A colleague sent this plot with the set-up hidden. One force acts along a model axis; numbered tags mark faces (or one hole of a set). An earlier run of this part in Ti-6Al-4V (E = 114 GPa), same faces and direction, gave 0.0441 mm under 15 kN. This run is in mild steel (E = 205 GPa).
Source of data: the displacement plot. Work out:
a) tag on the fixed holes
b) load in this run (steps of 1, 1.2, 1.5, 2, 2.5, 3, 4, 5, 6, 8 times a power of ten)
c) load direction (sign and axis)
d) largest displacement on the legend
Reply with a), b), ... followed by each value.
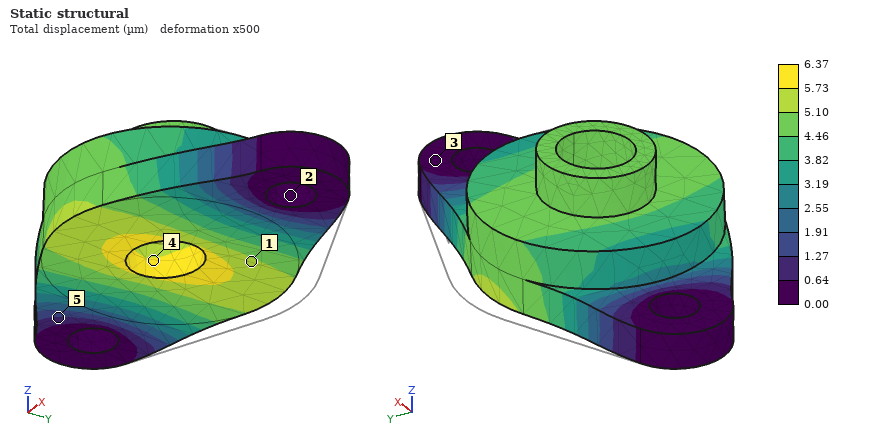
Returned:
a) 2
b) 4 kN
c) -Y
d) 6.37 µm
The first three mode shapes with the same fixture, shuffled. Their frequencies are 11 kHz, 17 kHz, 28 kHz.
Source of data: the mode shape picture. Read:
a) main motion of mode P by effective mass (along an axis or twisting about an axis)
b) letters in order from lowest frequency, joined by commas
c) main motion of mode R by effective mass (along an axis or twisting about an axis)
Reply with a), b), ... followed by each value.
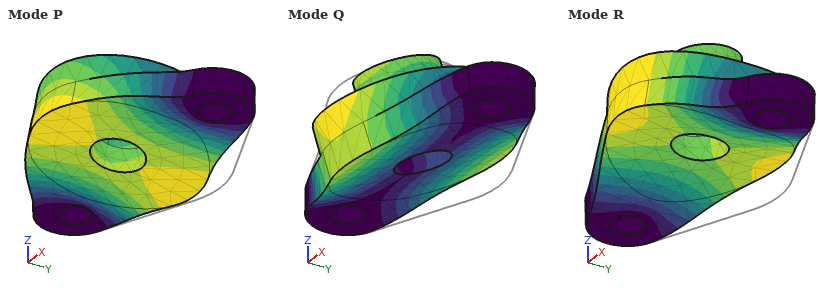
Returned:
a) along Y
b) Q, R, P
c) along Z
